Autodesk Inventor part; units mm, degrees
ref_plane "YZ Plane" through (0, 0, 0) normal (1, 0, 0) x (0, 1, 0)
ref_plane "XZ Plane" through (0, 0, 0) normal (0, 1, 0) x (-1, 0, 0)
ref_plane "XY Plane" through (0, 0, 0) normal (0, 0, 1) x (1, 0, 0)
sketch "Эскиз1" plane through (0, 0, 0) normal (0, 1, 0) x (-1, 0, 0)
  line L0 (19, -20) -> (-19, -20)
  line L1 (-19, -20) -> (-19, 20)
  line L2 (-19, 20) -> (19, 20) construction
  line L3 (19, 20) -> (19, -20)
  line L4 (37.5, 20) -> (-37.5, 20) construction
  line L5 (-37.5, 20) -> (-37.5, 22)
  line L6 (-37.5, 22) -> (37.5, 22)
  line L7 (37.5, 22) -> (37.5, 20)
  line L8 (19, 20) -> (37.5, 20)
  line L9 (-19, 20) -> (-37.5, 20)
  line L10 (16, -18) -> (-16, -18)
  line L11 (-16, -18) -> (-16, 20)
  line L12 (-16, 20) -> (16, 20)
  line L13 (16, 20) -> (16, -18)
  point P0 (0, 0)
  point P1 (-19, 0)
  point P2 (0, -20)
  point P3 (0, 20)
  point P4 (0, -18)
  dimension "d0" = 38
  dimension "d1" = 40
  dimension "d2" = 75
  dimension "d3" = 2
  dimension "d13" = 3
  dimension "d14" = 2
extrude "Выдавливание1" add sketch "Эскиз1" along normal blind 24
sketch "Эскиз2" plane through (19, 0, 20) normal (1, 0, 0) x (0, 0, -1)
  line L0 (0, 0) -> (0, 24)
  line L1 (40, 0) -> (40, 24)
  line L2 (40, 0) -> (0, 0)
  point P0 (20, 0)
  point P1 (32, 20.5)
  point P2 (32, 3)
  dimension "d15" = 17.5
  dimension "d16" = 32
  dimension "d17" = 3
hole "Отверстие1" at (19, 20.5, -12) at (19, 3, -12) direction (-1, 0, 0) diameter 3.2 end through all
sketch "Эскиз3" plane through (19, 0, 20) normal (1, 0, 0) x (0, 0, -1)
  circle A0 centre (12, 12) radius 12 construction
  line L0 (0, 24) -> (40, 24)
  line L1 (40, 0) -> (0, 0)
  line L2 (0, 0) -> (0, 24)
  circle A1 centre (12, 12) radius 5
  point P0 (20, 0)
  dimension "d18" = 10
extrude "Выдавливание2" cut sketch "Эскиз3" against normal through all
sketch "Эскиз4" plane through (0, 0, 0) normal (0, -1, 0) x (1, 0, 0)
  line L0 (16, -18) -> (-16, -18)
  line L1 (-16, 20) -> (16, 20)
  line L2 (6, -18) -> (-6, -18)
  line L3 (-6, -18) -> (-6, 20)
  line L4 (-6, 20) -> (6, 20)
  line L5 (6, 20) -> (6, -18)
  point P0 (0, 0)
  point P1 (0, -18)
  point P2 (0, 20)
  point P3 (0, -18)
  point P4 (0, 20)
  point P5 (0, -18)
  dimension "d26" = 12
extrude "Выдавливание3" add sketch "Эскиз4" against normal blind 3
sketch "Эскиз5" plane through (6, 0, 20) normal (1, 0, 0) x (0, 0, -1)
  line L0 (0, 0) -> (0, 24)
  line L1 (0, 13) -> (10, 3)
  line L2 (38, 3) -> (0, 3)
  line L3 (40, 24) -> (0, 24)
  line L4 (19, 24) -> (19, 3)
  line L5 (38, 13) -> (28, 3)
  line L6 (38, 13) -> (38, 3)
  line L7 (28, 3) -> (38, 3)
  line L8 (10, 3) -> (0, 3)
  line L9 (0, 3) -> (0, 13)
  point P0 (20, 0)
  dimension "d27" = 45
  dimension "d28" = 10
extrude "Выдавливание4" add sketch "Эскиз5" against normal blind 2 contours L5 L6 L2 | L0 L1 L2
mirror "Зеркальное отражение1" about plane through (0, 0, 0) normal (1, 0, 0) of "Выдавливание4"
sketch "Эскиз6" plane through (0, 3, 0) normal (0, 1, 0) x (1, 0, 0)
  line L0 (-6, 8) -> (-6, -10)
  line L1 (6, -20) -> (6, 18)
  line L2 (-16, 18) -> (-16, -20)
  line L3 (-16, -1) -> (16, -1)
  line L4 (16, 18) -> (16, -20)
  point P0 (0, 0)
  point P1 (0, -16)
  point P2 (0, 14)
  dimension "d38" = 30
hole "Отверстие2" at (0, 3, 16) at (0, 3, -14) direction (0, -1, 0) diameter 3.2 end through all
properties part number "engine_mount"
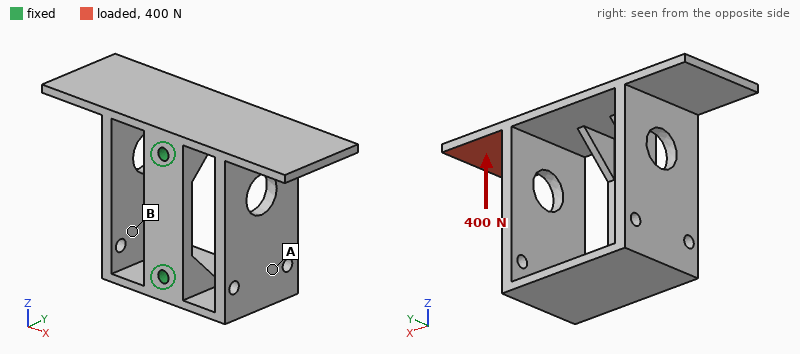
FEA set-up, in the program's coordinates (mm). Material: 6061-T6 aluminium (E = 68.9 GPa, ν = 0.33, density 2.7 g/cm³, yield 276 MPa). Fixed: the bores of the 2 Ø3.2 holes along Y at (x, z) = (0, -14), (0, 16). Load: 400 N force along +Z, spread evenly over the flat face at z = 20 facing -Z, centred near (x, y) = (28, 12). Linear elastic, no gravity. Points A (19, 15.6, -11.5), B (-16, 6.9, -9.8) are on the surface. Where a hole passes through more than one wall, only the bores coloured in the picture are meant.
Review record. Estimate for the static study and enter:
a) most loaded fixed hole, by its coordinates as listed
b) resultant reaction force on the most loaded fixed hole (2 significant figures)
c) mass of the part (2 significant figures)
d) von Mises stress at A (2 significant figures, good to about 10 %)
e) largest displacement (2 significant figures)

(0, -14)
420 N
33 g
32 MPa
0.64 mm
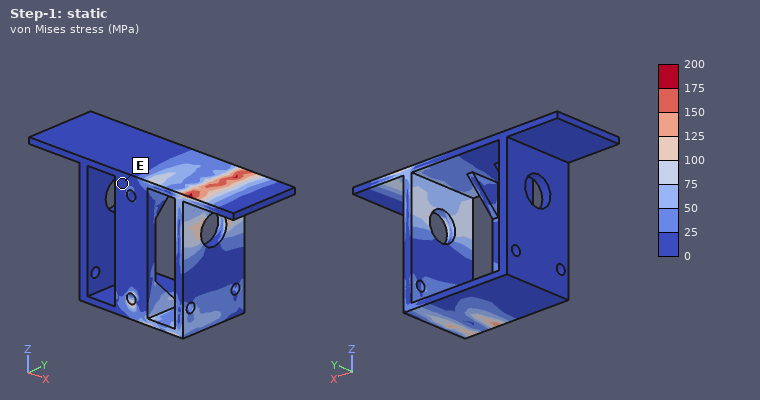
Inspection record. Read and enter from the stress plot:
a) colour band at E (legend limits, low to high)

0 to 25 MPa
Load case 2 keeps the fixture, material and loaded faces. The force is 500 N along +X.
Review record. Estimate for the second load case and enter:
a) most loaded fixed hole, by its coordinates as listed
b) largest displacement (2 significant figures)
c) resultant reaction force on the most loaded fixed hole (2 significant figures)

(0, 16)
0.18 mm
530 N
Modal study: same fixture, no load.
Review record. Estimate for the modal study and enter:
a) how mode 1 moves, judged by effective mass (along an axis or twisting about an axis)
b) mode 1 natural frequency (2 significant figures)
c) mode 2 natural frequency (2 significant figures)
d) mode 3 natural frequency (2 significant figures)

along X
1900 Hz
2700 Hz
2800 Hz
